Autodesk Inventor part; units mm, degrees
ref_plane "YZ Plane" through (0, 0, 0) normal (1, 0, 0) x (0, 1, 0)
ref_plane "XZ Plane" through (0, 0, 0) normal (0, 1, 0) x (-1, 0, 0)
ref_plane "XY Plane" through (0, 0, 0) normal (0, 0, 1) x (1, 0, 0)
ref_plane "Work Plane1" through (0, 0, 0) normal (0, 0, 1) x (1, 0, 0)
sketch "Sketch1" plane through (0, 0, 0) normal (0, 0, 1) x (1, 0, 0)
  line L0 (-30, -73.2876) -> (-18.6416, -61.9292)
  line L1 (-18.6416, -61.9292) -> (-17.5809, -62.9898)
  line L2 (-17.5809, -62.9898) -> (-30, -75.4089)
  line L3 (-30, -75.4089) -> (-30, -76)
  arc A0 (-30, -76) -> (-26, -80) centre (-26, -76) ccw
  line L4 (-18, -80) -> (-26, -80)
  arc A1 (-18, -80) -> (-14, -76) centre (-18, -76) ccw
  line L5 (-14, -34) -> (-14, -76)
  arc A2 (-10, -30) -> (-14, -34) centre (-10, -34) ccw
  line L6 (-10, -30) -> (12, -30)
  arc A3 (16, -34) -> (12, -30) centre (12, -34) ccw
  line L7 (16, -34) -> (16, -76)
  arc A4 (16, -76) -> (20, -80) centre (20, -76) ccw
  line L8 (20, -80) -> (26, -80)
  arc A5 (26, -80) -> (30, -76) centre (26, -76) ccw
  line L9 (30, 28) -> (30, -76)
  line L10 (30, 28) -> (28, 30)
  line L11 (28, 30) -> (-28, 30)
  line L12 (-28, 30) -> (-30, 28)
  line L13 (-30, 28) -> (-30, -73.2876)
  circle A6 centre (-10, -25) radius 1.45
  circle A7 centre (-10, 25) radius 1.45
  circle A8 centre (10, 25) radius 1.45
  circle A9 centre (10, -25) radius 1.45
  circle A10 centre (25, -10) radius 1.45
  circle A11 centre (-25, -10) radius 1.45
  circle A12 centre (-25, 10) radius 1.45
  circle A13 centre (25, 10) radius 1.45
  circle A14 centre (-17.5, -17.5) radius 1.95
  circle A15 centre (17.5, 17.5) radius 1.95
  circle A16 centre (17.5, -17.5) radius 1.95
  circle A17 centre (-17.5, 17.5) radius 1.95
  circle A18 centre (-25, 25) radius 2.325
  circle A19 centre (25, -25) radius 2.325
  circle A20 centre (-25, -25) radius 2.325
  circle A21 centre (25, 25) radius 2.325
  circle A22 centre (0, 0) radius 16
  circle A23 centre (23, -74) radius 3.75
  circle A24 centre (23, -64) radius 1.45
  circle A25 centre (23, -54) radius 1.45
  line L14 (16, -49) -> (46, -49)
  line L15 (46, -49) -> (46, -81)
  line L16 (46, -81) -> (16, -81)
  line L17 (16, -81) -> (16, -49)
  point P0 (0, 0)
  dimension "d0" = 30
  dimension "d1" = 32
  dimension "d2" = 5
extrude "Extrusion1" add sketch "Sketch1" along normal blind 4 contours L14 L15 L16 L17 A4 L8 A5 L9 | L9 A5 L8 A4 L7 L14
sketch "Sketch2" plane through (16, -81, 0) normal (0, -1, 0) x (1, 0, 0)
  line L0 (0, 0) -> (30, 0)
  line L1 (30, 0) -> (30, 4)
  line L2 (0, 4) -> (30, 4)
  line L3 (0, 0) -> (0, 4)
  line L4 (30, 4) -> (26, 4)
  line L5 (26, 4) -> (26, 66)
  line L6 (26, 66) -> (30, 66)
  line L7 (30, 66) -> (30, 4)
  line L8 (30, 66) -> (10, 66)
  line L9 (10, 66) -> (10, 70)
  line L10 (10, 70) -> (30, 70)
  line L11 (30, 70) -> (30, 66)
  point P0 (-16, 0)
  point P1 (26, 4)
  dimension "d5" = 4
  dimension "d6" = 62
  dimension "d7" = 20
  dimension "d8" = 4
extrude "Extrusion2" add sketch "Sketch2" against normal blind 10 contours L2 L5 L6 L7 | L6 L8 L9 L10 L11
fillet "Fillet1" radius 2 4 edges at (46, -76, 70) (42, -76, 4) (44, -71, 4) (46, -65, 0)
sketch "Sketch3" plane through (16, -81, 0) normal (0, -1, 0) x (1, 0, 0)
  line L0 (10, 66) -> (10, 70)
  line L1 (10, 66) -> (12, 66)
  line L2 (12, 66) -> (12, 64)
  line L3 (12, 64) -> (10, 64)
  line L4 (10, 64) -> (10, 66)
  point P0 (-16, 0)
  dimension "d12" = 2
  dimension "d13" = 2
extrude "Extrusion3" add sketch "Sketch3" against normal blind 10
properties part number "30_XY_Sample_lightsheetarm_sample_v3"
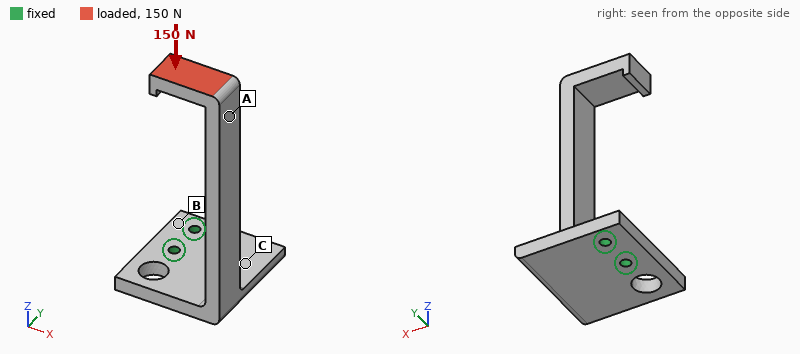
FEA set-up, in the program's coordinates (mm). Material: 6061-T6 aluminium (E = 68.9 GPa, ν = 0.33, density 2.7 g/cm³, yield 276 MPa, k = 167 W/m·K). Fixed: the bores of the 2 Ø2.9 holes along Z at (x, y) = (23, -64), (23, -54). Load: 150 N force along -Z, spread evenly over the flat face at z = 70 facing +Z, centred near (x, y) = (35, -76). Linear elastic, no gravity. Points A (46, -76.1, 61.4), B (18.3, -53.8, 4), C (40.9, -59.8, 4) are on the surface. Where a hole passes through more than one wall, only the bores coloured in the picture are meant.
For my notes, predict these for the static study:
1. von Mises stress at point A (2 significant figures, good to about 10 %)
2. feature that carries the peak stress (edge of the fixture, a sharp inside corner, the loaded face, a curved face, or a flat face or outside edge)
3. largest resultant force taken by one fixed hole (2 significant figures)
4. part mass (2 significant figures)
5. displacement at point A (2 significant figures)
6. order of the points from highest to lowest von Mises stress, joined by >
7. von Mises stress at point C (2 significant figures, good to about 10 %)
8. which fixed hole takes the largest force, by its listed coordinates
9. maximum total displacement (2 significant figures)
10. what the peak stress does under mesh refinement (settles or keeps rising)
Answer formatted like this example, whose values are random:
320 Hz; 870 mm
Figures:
45 MPa; edge of the fixture; 230 N; 19 g; 0.57 mm; A > C > B; 12 MPa; (23, -64); 0.91 mm; keeps rising
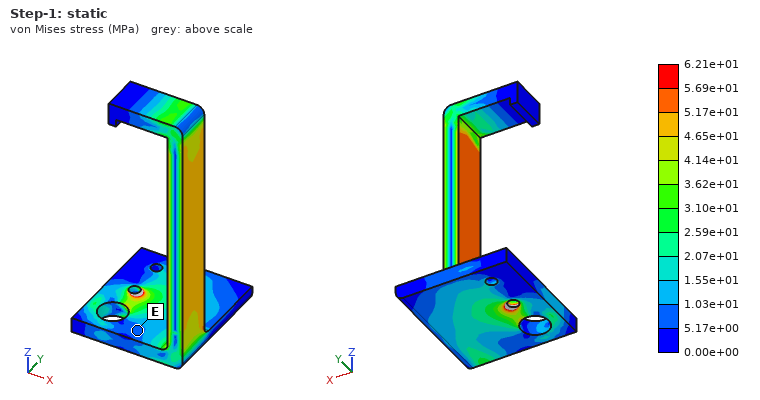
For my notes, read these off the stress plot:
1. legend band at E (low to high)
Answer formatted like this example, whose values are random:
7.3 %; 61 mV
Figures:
5.17e+00 to 1.03e+01 MPa
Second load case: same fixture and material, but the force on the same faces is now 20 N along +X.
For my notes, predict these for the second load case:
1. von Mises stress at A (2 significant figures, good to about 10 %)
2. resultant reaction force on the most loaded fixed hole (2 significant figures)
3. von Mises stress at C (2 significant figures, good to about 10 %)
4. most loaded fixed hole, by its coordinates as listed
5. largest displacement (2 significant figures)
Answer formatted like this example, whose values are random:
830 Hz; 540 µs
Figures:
6.4 MPa; 39 N; 12 MPa; (23, -64); 0.81 mm
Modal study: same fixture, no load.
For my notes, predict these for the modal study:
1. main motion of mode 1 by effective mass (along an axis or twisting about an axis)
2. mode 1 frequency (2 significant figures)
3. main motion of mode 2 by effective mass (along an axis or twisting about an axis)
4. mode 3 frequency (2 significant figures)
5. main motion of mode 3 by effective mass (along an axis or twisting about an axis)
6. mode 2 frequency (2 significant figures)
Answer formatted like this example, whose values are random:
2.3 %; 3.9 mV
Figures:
along X; 420 Hz; along Y; 2000 Hz; along Z; 650 Hz
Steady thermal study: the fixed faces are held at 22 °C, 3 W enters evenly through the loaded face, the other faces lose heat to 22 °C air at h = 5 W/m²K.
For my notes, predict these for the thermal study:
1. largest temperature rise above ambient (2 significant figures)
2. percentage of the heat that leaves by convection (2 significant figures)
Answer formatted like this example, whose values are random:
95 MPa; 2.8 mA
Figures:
36 K; 8.5 %
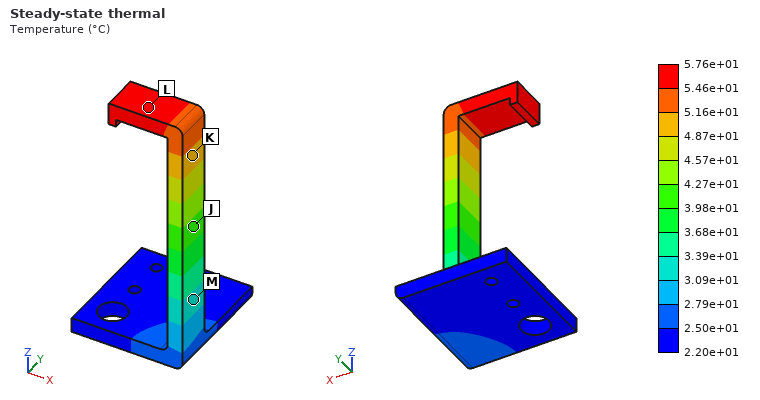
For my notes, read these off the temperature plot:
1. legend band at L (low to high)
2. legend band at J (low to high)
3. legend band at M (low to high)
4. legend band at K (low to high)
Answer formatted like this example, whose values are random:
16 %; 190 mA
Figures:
5.46e+01 to 5.76e+01 °C; 3.98e+01 to 4.27e+01 °C; 3.09e+01 to 3.39e+01 °C; 4.87e+01 to 5.16e+01 °C
